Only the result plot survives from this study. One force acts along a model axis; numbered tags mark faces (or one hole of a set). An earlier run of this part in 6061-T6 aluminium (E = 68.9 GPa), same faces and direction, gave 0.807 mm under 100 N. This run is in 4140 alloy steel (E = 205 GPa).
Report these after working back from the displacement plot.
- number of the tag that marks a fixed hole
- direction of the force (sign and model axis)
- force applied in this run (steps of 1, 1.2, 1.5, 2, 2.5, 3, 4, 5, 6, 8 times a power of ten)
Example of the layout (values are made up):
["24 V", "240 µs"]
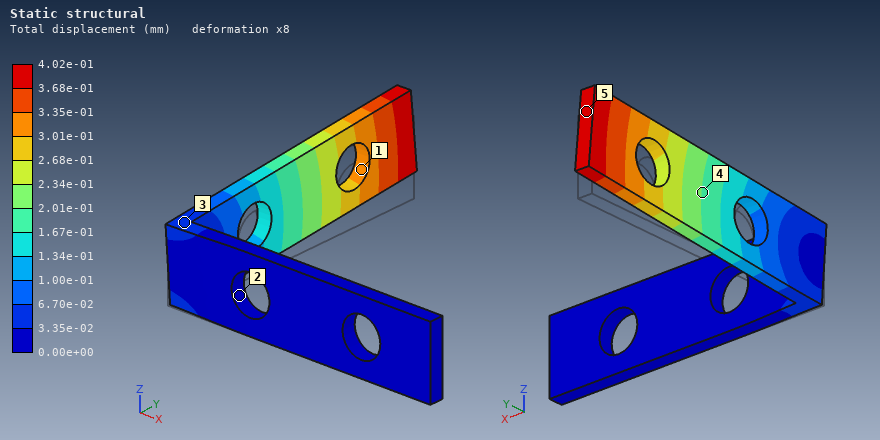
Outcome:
["2", "+Z", "150 N"]
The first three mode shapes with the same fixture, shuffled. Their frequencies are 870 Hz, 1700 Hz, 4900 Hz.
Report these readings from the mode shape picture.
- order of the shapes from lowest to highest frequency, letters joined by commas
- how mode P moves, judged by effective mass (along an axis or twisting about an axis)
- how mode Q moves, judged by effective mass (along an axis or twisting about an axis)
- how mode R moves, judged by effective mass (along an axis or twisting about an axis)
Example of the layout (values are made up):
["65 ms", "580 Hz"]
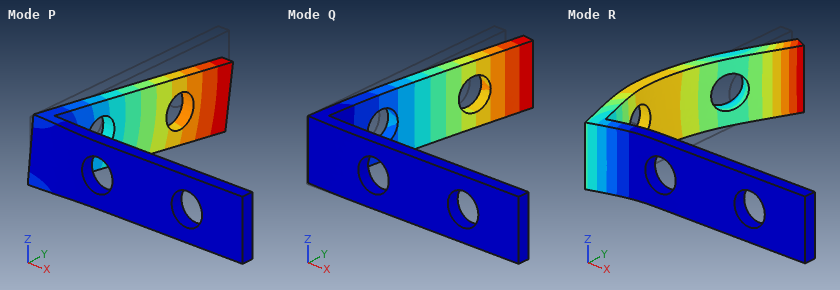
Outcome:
["Q, P, R", "along Z", "along X", "along Y"]
